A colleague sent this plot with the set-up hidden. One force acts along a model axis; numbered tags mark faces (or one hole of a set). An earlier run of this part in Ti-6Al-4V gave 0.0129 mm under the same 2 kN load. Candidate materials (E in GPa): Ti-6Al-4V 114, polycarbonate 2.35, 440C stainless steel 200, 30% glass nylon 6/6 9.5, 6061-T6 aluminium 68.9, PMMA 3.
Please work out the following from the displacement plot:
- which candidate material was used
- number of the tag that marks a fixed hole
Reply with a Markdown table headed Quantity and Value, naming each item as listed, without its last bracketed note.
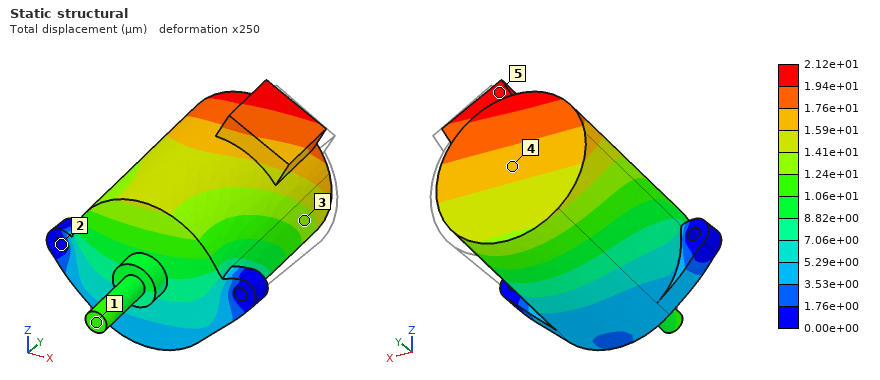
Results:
| Quantity | Value |
|---|---|
| which candidate material was used | 6061-T6 aluminium |
| number of the tag that marks a fixed hole | 2 |
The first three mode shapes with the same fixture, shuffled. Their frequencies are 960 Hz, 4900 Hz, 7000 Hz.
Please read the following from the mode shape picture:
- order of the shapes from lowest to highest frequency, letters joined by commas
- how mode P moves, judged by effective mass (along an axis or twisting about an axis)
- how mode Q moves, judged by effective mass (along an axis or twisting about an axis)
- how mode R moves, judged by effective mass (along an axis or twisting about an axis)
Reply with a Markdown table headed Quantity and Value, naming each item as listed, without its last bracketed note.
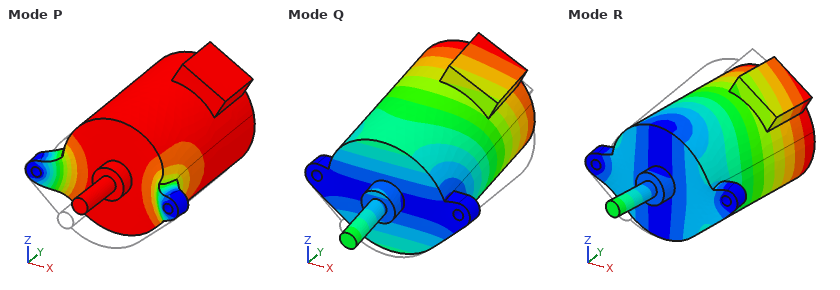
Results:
| Quantity | Value |
|---|---|
| order of the shapes from lowest to highest frequency, letters joined by commas | Q, R, P |
| how mode P moves, judged by effective mass | along Y |
| how mode Q moves, judged by effective mass | along Z |
| how mode R moves, judged by effective mass | along X |
